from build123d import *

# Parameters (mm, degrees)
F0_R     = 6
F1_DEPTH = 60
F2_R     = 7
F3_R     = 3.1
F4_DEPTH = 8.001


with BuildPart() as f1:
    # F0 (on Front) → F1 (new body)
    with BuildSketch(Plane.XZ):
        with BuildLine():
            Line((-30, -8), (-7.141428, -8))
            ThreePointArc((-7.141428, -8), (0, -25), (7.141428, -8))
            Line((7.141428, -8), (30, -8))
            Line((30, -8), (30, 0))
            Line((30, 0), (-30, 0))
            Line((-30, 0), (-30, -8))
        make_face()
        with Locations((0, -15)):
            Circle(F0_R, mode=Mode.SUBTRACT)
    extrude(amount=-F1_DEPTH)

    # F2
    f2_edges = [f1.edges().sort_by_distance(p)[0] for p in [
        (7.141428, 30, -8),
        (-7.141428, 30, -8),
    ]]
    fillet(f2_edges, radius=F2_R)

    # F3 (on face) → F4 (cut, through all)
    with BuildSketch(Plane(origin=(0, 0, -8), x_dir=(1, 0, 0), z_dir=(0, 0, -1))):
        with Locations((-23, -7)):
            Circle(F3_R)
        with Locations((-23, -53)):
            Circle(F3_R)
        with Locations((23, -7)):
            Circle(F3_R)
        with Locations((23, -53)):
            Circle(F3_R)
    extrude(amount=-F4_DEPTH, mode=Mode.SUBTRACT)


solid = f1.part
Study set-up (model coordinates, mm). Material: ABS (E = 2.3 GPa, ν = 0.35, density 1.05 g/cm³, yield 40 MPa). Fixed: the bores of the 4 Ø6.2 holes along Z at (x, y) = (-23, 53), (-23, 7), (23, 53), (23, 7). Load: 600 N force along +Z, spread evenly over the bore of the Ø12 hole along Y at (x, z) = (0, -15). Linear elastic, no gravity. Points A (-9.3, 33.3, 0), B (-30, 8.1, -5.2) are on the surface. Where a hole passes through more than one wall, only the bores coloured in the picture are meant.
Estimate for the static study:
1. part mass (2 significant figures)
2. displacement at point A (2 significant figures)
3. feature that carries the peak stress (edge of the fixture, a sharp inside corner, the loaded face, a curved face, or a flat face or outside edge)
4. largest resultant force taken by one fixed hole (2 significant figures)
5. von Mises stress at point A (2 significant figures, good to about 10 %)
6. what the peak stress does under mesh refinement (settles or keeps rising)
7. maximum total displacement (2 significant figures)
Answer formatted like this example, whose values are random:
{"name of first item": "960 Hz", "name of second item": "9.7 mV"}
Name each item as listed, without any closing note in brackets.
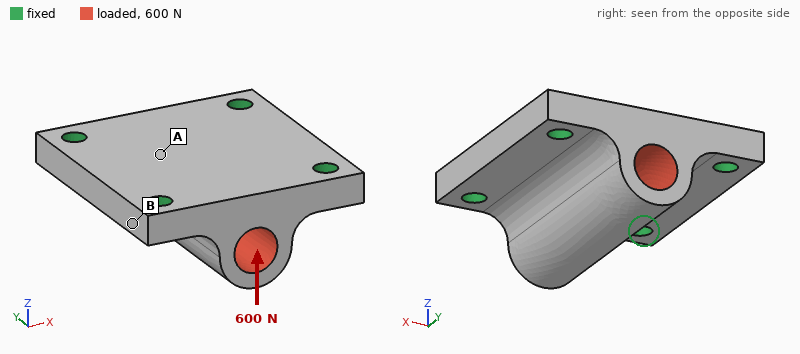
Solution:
{"part mass": "42 g", "displacement at point A": "38 µm", "feature that carries the peak stress": "edge of the fixture", "largest resultant force taken by one fixed hole": "160 N", "von Mises stress at point A": "1.2 MPa", "what the peak stress does under mesh refinement": "keeps rising", "maximum total displacement": "44 µm"}
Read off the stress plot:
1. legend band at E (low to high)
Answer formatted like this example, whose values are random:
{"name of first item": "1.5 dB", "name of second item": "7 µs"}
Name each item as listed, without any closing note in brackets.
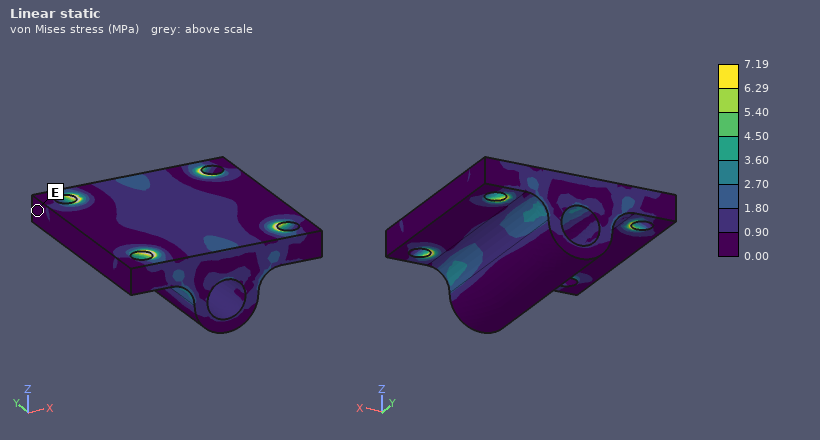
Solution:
{"legend band at E": "0.00 to 0.90 MPa"}
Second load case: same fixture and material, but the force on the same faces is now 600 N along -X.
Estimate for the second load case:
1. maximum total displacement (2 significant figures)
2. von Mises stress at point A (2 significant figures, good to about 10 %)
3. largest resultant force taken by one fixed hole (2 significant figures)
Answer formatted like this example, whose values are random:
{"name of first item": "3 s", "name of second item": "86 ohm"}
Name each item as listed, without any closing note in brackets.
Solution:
{"maximum total displacement": "41 µm", "von Mises stress at point A": "0.38 MPa", "largest resultant force taken by one fixed hole": "180 N"}
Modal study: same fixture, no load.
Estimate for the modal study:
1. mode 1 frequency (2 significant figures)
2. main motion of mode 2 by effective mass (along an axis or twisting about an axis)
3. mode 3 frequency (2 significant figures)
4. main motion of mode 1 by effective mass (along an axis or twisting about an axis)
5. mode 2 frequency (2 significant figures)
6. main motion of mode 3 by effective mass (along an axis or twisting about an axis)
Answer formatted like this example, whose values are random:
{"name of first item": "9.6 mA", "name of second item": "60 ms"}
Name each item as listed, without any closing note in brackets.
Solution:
{"mode 1 frequency": "3700 Hz", "main motion of mode 2 by effective mass": "along Y", "mode 3 frequency": "5200 Hz", "main motion of mode 1 by effective mass": "along Z", "mode 2 frequency": "4500 Hz", "main motion of mode 3 by effective mass": "along X"}
